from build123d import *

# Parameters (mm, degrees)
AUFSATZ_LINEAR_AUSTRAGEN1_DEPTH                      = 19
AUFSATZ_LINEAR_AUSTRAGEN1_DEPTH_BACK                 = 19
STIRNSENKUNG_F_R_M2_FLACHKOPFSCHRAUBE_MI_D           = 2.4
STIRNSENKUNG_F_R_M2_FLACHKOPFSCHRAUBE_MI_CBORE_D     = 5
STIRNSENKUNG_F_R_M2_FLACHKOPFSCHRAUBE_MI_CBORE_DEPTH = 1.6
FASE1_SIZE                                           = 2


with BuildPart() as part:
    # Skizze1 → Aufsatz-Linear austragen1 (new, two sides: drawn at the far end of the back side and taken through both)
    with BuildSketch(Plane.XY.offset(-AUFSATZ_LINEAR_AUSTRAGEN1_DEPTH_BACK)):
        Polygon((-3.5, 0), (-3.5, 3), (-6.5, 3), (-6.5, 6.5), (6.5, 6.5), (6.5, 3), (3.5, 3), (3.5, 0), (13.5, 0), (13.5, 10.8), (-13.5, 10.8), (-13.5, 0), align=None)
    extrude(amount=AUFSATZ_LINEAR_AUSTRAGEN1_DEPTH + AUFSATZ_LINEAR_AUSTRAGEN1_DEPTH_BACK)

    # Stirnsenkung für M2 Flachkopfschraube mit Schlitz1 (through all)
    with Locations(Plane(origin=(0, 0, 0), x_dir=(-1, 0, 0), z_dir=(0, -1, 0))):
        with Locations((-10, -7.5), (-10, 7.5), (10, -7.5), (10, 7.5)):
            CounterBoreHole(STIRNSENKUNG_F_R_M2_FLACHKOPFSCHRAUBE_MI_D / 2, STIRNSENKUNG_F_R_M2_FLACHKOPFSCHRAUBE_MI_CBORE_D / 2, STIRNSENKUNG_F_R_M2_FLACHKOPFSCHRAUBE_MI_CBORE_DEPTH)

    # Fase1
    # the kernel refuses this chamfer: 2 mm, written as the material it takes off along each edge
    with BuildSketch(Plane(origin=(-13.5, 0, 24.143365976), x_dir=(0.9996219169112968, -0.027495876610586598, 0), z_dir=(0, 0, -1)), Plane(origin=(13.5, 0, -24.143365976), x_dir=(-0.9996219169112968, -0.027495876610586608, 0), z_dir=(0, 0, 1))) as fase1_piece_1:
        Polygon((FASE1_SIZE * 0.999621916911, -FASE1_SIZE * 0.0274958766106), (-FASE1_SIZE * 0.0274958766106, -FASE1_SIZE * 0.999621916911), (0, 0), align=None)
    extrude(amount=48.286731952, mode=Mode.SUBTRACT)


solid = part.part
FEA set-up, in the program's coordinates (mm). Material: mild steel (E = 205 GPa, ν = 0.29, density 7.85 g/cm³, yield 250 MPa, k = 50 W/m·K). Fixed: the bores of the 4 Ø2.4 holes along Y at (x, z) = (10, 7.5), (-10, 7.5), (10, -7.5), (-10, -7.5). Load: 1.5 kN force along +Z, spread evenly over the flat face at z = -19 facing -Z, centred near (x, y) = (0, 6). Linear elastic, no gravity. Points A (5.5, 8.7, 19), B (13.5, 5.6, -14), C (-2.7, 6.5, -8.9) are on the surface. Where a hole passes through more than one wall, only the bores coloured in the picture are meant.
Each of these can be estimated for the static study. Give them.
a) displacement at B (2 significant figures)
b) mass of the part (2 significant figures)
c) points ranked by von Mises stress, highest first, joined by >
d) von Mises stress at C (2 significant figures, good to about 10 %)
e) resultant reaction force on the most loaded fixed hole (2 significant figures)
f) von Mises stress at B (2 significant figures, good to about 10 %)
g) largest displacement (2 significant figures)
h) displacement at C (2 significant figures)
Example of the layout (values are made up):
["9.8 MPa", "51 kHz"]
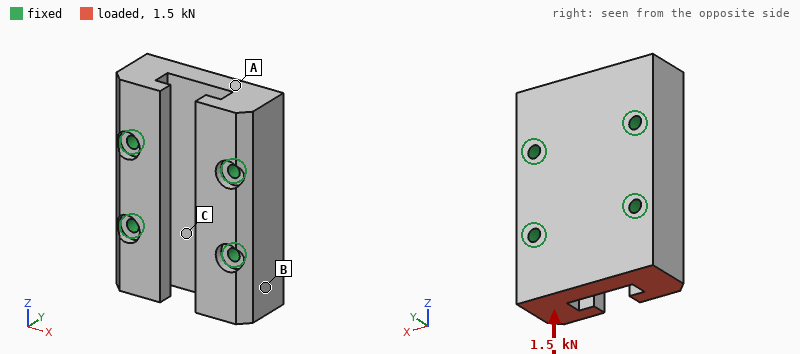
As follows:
["0.26 µm", "64 g", "B > C > A", "4.1 MPa", "640 N", "7.2 MPa", "0.58 µm", "0.24 µm"]
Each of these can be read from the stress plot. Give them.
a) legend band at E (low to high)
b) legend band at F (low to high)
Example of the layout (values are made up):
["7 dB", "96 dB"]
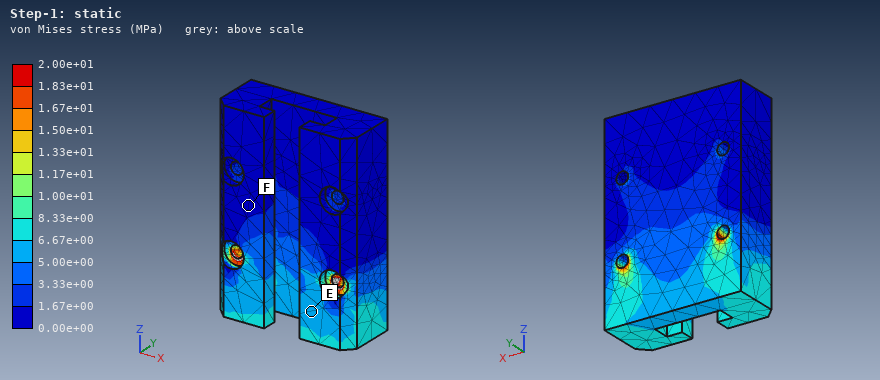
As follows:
["5.00e+00 to 6.67e+00 MPa", "0.00e+00 to 1.67e+00 MPa"]
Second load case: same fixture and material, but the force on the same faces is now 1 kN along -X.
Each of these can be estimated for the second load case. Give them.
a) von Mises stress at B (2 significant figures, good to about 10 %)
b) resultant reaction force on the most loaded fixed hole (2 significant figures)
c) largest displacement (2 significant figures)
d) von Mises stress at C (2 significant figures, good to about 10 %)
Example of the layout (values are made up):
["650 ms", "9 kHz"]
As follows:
["12 MPa", "700 N", "2.7 µm", "11 MPa"]
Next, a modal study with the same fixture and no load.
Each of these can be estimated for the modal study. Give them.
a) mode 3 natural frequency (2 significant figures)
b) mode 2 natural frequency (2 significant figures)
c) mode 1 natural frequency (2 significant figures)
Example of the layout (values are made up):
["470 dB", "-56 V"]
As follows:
["40 kHz", "32 kHz", "32 kHz"]
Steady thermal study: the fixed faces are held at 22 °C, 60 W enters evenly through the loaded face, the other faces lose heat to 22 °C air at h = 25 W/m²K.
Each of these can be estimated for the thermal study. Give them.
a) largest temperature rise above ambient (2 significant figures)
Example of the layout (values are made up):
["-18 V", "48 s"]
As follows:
["70 K"]
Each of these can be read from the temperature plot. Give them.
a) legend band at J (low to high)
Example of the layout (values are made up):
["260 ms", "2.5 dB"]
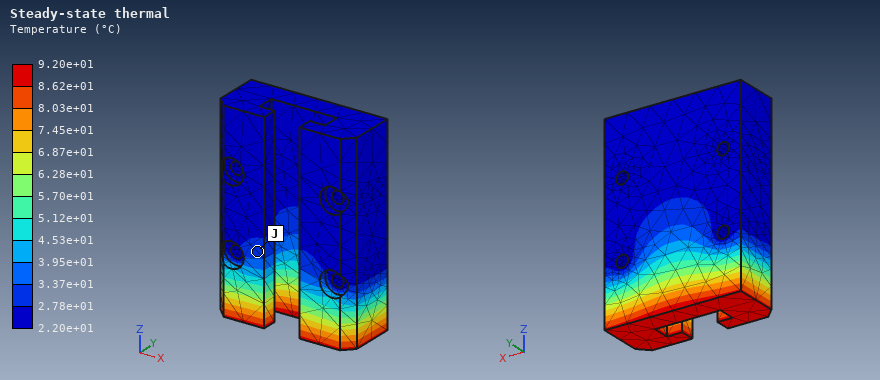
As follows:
["2.78e+01 to 3.37e+01 °C"]
